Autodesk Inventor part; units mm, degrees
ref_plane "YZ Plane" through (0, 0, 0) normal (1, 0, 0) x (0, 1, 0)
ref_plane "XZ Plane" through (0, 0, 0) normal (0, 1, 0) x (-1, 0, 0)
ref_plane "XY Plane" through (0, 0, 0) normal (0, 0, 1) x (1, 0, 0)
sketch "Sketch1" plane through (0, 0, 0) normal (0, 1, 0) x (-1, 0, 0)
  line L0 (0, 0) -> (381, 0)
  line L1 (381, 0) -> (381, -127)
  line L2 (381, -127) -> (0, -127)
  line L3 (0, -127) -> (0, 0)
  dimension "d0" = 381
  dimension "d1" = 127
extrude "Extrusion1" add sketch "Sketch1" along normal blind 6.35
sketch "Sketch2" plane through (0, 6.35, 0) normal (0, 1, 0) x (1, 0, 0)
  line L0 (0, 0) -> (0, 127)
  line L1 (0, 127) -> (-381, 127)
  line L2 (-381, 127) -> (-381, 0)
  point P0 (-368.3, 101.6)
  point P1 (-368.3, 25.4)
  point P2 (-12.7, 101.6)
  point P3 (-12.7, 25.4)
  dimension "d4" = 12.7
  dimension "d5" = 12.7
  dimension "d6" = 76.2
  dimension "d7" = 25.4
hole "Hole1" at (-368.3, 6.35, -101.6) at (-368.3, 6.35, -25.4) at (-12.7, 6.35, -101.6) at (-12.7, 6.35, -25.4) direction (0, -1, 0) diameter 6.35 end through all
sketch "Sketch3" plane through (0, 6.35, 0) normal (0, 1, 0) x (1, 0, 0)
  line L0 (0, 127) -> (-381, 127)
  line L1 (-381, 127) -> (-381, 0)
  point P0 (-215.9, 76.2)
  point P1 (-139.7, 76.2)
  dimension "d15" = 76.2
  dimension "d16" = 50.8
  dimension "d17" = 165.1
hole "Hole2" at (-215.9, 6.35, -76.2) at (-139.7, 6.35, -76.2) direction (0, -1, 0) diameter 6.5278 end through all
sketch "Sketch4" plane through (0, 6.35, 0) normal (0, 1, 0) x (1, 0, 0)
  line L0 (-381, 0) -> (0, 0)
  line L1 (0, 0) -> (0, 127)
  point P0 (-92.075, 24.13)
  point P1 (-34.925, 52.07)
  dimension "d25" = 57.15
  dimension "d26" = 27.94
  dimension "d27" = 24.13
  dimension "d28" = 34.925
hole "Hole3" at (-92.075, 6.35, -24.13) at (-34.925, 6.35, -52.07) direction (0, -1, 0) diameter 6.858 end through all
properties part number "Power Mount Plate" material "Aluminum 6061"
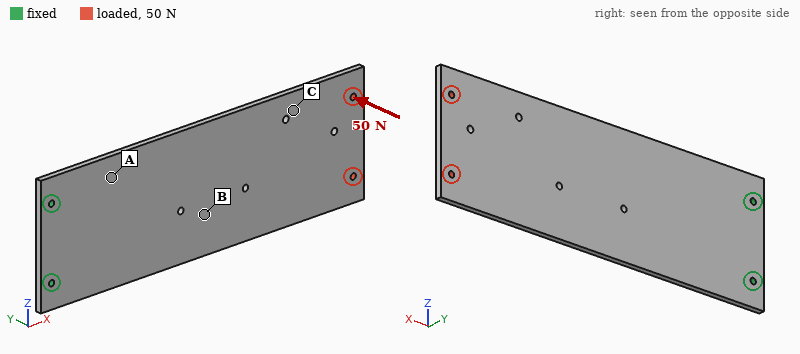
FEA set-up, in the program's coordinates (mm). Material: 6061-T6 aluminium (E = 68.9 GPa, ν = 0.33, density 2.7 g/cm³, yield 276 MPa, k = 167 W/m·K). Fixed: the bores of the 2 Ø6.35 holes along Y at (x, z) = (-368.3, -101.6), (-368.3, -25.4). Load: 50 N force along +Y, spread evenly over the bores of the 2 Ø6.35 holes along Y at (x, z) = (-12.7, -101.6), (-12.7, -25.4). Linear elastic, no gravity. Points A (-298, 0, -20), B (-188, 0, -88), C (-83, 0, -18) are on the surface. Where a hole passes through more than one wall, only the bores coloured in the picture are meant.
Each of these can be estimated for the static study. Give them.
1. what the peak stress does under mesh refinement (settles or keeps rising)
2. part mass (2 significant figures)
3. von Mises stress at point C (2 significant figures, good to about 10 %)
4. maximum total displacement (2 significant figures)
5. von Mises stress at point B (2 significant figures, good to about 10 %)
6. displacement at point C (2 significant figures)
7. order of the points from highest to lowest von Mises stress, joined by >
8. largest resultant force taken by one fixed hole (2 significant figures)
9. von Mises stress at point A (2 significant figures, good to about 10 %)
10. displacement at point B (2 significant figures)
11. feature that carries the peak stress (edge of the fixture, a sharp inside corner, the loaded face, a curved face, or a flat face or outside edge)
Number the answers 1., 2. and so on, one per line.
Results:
1. keeps rising
2. 830 g
3. 4.1 MPa
4. 4.4 mm
5. 10 MPa
6. 3.0 mm
7. A > B > C
8. 25 N
9. 16 MPa
10. 1.4 mm
11. edge of the fixture
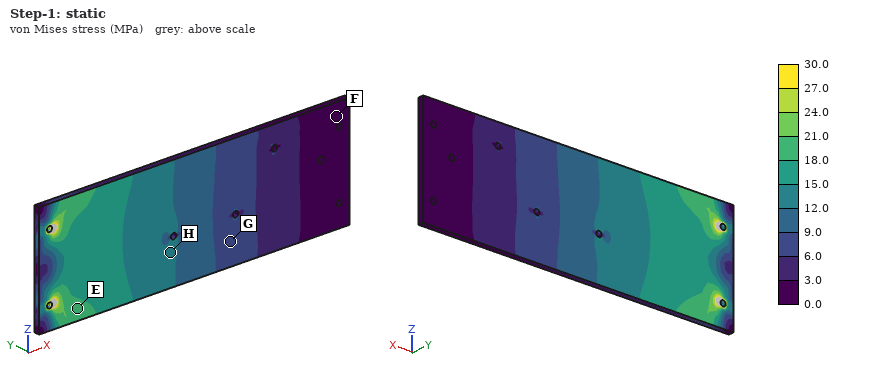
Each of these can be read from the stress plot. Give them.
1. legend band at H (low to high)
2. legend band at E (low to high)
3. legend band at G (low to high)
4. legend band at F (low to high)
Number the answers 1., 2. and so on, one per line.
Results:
1. 12.0 to 15.0 MPa
2. 18.0 to 21.0 MPa
3. 6.0 to 9.0 MPa
4. 0.0 to 3.0 MPa
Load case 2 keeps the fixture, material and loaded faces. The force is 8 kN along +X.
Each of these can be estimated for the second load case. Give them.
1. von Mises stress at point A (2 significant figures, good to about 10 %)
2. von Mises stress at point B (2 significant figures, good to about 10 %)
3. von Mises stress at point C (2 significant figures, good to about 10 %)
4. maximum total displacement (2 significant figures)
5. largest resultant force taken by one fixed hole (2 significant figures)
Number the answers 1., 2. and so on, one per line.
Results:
1. 10 MPa
2. 9.8 MPa
3. 11 MPa
4. 64 µm
5. 4.0 kN
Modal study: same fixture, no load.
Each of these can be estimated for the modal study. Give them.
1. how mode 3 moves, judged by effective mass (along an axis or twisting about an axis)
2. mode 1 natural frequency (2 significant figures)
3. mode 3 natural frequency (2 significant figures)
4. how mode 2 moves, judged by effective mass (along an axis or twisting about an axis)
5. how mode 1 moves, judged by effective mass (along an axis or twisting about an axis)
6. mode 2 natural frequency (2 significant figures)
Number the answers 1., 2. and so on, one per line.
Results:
1. along Y
2. 37 Hz
3. 230 Hz
4. twisting about X
5. along Y
6. 220 Hz
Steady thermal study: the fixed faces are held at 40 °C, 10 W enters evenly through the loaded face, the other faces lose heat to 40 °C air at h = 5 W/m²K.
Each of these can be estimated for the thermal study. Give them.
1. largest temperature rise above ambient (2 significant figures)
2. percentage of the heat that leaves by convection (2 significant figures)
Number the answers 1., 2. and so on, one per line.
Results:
1. 20 K
2. 45 %
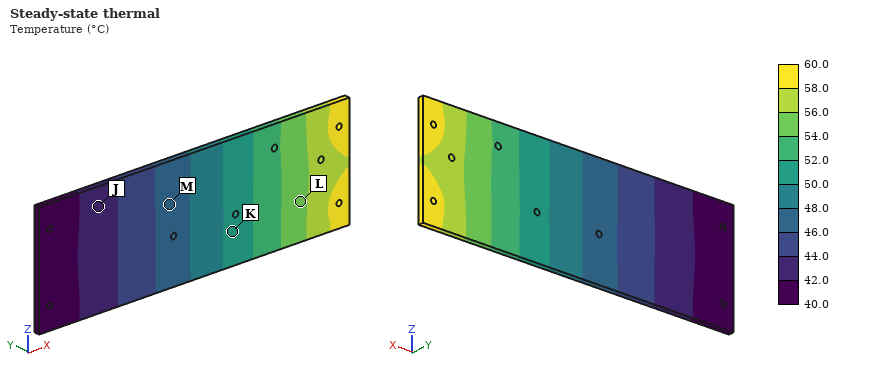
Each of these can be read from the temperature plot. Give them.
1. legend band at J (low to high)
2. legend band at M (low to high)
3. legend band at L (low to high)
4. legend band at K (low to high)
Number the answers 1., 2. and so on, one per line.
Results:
1. 42.0 to 44.0 °C
2. 46.0 to 48.0 °C
3. 54.0 to 56.0 °C
4. 50.0 to 52.0 °C
